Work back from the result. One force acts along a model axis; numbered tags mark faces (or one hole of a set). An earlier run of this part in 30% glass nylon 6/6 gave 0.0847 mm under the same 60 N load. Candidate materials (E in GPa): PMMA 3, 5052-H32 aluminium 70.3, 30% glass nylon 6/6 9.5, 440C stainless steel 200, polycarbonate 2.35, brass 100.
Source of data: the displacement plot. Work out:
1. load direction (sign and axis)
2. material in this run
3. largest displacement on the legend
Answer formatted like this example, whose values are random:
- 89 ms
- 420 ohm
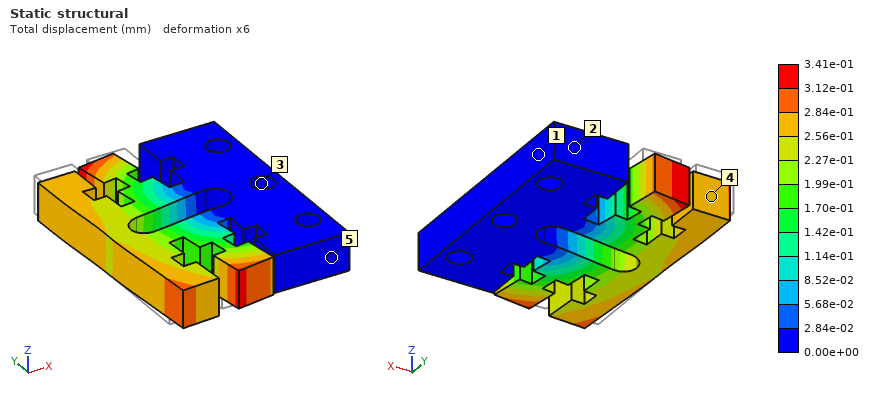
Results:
- -Y
- polycarbonate
- 3.41e-01 mm
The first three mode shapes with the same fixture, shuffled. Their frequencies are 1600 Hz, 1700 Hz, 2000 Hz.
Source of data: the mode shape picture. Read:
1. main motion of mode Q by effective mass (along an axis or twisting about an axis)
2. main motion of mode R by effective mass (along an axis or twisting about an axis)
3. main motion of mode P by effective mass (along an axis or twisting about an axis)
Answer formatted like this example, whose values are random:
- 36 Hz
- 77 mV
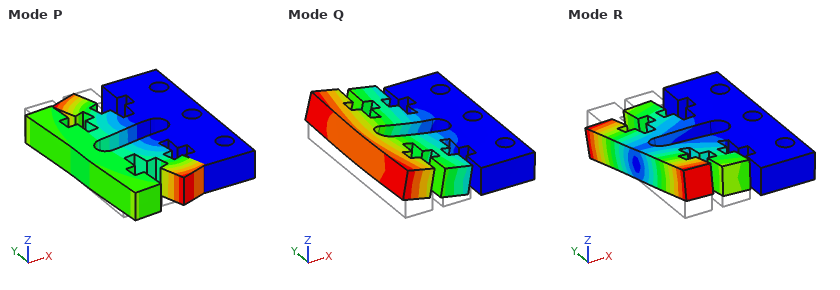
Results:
- along Z
- twisting about X
- along Y
